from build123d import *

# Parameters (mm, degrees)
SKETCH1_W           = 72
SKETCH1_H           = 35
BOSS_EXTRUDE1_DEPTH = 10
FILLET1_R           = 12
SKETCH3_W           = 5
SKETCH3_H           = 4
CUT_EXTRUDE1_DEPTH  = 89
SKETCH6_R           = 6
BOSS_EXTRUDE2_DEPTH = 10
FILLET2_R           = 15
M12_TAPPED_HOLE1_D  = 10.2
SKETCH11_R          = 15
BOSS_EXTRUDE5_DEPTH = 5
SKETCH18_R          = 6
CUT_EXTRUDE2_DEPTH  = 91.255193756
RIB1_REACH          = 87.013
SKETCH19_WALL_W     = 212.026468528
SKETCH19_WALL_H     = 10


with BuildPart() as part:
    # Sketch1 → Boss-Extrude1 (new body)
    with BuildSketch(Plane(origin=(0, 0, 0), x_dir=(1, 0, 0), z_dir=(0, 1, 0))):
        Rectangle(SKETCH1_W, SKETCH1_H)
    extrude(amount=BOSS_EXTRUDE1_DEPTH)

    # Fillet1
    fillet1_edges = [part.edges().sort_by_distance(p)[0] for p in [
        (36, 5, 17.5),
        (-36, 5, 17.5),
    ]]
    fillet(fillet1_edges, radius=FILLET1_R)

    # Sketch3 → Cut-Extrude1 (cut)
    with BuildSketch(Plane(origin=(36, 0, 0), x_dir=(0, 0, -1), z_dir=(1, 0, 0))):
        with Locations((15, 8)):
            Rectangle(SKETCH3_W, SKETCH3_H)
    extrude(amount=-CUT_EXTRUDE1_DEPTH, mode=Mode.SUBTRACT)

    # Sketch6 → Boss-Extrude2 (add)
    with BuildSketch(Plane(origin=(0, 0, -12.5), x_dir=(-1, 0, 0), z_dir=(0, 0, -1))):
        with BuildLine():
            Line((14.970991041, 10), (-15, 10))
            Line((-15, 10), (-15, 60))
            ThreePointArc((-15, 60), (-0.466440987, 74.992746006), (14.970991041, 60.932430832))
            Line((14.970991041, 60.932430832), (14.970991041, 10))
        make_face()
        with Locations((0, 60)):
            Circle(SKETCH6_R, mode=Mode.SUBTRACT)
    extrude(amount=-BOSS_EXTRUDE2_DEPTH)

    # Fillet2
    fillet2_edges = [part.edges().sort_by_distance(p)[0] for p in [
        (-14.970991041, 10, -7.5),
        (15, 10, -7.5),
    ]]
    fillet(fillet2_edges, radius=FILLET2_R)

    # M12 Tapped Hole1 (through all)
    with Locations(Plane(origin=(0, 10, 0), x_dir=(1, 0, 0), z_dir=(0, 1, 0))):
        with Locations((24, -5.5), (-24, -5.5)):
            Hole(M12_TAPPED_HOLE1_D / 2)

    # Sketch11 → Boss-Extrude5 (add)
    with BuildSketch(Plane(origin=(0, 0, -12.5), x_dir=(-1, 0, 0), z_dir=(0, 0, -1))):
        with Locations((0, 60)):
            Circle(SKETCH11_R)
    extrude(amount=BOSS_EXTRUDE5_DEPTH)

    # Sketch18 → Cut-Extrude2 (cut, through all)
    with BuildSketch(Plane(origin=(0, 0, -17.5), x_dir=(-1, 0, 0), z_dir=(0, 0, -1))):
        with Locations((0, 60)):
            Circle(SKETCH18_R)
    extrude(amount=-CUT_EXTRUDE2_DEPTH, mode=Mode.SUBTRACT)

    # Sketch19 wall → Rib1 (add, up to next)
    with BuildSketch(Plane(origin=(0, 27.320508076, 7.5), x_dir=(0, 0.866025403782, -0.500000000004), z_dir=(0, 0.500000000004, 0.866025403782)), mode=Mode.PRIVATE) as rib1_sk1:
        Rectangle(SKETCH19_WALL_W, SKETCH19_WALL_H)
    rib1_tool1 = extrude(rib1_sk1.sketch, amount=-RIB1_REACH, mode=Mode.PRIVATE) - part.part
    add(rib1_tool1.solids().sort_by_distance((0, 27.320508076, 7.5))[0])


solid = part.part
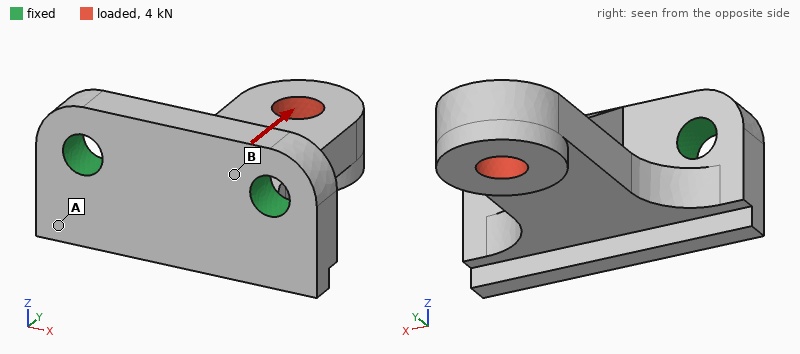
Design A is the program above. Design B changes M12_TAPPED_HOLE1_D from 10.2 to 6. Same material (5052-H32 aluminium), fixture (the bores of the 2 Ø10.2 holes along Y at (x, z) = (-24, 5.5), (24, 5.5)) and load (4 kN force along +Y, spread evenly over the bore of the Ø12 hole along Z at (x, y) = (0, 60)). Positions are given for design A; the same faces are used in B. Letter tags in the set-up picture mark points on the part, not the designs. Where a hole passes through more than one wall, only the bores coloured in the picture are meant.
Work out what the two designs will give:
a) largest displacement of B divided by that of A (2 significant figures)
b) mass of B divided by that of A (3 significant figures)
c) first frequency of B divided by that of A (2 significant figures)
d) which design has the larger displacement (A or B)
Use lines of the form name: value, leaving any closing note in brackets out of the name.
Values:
largest displacement of B divided by that of A: 1.3
mass of B divided by that of A: 1.02
first frequency of B divided by that of A: 0.90
which design has the larger displacement: B
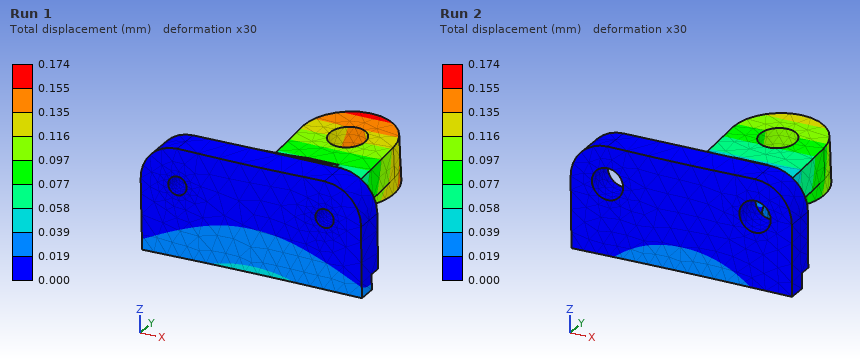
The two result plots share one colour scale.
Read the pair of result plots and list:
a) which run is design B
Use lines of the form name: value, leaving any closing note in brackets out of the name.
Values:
which run is design B: Run 1
